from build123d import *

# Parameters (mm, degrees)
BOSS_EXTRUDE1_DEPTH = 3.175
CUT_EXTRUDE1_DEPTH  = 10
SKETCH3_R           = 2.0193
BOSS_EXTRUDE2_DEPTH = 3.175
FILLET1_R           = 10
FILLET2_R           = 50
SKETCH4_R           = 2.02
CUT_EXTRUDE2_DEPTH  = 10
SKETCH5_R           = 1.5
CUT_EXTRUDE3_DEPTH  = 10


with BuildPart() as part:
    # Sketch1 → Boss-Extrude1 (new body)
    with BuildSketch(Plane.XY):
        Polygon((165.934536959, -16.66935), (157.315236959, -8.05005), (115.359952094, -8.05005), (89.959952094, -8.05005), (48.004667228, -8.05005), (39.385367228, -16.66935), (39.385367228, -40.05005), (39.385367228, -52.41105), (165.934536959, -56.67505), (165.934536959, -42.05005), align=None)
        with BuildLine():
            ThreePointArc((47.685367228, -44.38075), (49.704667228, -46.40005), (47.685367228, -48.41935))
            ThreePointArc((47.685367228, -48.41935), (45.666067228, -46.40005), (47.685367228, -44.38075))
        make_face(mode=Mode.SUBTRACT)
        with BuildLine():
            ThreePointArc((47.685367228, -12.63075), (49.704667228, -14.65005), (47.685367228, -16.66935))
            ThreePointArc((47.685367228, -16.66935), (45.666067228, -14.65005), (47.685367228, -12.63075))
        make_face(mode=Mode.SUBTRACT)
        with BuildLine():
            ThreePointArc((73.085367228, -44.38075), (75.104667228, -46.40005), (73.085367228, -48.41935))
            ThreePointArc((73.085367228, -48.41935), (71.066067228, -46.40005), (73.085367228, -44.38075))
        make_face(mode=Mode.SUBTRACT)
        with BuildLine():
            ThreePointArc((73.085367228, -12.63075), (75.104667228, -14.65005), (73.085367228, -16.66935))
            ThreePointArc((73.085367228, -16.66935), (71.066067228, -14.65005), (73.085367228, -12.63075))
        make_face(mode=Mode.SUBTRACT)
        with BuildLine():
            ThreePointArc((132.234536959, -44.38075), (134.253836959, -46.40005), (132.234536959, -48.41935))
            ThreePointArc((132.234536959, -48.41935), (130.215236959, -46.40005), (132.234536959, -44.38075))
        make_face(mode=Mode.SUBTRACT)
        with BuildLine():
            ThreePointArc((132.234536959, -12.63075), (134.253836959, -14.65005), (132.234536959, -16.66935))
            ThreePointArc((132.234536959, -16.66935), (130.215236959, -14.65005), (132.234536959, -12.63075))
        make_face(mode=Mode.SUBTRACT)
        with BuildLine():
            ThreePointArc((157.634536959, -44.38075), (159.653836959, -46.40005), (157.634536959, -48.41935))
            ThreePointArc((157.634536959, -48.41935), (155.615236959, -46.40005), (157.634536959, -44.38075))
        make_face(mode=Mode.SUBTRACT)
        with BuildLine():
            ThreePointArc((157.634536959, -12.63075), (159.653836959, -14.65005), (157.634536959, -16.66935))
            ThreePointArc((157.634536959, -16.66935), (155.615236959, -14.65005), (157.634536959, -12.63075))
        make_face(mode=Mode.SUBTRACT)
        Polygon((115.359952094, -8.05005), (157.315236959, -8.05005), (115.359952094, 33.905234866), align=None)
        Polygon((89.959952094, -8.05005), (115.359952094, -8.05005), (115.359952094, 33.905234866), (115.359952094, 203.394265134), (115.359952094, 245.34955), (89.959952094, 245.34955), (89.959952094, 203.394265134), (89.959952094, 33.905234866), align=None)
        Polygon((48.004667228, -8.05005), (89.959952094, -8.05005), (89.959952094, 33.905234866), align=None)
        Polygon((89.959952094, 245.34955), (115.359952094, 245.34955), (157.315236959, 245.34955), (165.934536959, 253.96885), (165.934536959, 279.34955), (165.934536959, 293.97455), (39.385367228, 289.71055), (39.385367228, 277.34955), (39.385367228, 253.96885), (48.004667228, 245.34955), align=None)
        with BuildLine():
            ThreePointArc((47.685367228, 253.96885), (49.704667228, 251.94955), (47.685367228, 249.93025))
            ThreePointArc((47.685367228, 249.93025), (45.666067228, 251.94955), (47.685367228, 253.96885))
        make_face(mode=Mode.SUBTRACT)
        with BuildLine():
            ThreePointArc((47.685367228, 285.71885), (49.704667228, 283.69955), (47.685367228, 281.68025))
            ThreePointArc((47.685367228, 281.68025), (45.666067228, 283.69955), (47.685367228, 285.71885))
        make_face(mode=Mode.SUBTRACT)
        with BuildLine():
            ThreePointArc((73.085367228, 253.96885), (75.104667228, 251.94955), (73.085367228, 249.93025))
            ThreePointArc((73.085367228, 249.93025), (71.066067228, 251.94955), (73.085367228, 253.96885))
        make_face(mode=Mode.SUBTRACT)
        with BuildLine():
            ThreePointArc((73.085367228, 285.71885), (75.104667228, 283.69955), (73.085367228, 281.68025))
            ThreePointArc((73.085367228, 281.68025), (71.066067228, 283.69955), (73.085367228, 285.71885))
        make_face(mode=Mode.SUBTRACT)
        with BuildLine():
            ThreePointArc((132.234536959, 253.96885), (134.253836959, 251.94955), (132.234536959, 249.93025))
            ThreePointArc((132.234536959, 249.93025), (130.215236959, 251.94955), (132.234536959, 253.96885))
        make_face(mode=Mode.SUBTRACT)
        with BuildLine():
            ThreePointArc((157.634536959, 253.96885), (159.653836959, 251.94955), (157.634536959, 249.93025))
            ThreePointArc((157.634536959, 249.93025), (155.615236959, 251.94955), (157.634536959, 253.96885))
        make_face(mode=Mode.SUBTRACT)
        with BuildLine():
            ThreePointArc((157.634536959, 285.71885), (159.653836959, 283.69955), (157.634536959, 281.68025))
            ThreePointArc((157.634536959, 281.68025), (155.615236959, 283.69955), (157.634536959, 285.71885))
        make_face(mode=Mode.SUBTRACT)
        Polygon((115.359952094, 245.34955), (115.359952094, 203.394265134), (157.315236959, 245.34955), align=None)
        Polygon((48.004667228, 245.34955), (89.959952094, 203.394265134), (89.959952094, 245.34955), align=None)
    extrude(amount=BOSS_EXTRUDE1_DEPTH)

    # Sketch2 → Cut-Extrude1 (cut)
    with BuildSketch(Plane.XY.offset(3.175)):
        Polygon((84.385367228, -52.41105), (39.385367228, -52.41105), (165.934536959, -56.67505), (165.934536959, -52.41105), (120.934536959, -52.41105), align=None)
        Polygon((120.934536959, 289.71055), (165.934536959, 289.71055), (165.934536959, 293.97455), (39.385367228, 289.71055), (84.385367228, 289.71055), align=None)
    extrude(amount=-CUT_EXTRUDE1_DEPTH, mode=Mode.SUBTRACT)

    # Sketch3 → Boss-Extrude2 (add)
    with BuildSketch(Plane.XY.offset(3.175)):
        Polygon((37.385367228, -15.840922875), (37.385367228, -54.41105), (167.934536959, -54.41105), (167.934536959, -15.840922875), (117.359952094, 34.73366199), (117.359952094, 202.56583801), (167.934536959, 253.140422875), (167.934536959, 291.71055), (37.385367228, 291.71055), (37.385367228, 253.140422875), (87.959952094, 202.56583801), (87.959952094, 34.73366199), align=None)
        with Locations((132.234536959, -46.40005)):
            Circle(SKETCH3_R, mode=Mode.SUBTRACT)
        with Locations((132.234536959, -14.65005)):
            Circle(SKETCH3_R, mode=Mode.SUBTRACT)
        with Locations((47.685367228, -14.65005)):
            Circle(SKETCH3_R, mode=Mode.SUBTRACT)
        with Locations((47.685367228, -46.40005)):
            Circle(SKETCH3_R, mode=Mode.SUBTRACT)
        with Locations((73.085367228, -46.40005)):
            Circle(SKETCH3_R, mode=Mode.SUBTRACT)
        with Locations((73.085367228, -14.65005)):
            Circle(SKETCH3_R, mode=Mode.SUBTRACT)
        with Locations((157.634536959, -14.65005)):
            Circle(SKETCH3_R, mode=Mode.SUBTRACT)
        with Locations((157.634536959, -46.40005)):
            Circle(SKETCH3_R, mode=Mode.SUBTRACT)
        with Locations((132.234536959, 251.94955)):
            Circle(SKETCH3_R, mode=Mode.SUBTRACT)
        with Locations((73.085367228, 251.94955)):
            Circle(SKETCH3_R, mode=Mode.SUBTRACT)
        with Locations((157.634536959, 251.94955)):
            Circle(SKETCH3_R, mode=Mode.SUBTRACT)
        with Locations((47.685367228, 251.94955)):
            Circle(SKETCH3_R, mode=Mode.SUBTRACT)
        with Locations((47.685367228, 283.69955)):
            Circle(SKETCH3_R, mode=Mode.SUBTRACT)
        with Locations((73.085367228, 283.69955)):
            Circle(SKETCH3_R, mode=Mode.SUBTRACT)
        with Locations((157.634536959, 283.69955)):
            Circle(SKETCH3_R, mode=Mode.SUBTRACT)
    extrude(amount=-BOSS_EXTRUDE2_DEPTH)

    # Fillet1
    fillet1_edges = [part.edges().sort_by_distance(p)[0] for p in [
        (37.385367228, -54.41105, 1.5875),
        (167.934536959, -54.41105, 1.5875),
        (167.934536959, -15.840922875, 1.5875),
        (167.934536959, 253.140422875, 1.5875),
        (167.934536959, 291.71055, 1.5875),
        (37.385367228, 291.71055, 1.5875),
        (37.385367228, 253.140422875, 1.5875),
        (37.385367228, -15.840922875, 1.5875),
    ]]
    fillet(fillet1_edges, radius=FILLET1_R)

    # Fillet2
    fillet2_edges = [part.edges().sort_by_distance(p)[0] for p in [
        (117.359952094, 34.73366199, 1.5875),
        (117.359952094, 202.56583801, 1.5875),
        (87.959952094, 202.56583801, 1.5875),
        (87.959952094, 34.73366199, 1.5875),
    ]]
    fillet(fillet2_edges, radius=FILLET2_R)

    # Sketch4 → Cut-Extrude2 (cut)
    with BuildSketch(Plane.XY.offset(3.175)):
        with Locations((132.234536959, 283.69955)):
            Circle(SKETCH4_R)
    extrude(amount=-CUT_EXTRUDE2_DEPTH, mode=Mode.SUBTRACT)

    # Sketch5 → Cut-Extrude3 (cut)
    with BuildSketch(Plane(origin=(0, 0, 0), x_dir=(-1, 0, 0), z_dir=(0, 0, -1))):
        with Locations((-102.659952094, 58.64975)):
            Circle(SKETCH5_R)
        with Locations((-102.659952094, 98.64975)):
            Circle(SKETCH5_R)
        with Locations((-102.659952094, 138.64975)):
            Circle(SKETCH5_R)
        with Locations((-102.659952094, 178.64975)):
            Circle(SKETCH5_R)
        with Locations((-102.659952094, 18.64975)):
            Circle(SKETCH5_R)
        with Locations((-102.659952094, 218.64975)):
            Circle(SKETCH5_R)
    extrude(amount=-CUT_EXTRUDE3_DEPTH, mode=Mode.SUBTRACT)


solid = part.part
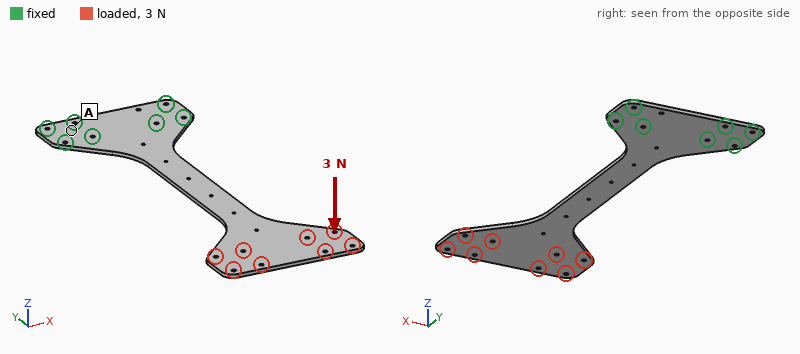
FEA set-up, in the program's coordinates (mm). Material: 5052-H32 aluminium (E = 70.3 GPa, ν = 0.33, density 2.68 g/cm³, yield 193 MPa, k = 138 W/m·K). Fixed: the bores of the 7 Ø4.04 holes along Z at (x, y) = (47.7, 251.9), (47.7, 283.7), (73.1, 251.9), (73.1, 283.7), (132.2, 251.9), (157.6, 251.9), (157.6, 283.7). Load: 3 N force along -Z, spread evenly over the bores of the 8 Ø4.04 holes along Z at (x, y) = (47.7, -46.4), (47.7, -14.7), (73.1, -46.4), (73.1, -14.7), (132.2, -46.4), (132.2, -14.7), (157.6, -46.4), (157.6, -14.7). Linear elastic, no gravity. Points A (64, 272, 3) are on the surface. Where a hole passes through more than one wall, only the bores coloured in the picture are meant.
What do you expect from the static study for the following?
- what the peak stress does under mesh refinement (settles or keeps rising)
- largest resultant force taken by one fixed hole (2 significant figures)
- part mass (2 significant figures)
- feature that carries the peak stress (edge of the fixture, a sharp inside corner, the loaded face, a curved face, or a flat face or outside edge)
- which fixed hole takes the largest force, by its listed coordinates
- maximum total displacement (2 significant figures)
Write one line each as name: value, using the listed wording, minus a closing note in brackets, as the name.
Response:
what the peak stress does under mesh refinement: keeps rising
largest resultant force taken by one fixed hole: 10 N
part mass: 200 g
feature that carries the peak stress: a sharp inside corner
which fixed hole takes the largest force, by its listed coordinates: (73.1, 251.9)
maximum total displacement: 3.5 mm
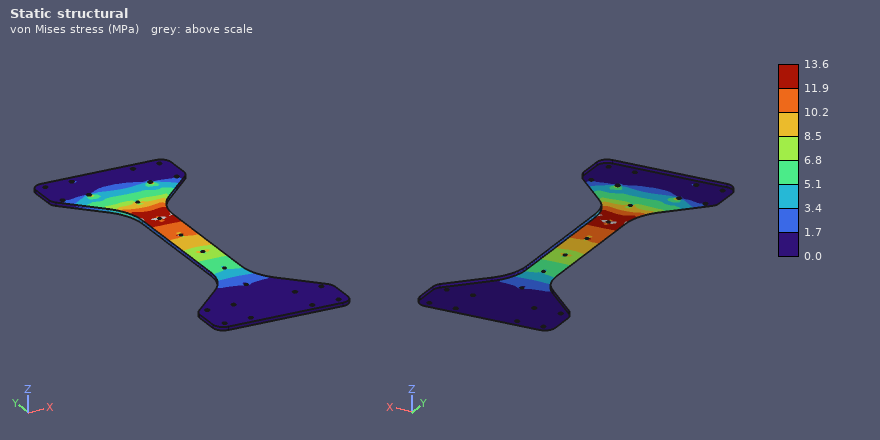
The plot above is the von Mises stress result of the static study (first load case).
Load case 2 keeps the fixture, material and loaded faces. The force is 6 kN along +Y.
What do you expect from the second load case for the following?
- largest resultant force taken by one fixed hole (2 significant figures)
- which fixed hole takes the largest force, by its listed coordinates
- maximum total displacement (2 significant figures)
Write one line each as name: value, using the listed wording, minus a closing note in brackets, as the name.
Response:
largest resultant force taken by one fixed hole: 2.2 kN
which fixed hole takes the largest force, by its listed coordinates: (132.2, 251.9)
maximum total displacement: 0.23 mm
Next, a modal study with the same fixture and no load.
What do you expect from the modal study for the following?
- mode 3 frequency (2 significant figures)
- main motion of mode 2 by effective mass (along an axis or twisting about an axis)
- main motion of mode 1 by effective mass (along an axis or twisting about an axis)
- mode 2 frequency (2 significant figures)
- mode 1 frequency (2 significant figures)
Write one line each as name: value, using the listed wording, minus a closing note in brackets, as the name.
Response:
mode 3 frequency: 170 Hz
main motion of mode 2 by effective mass: twisting about Y
main motion of mode 1 by effective mass: along Z
mode 2 frequency: 110 Hz
mode 1 frequency: 19 Hz
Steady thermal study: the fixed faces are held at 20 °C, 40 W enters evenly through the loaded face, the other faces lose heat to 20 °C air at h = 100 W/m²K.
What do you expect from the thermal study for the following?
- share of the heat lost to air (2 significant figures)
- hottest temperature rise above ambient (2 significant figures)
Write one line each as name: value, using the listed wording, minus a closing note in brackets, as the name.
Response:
share of the heat lost to air: 100 %
hottest temperature rise above ambient: 30 K
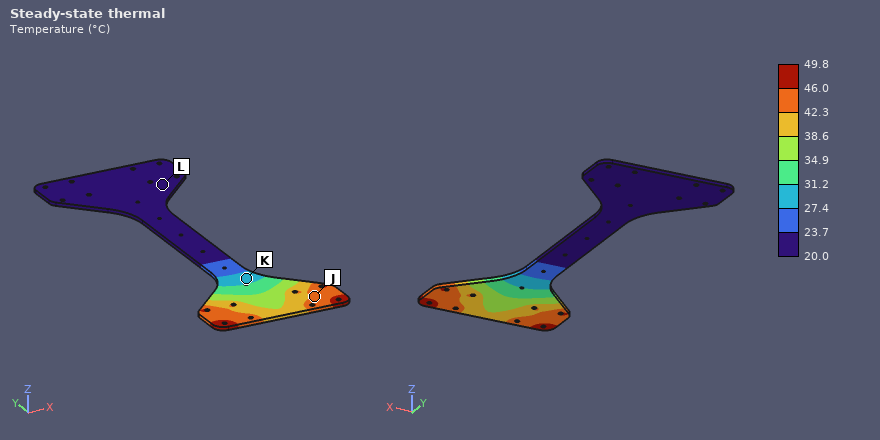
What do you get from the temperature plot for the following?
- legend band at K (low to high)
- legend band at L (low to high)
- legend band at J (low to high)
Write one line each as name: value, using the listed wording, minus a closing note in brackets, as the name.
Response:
legend band at K: 27.4 to 31.2 °C
legend band at L: 20.0 to 23.7 °C
legend band at J: 42.3 to 46.0 °C
